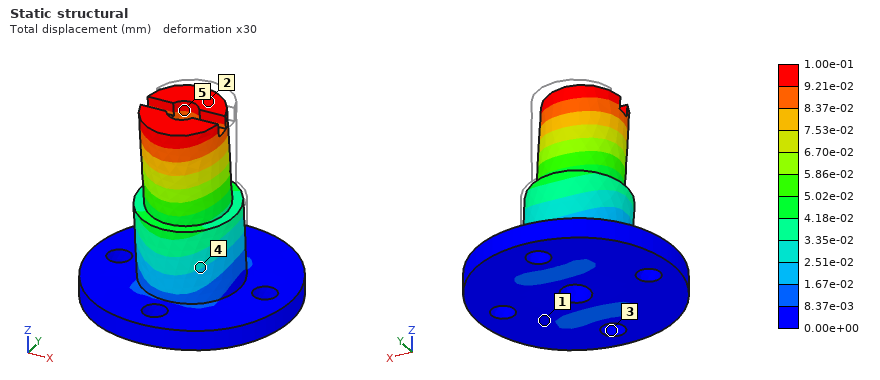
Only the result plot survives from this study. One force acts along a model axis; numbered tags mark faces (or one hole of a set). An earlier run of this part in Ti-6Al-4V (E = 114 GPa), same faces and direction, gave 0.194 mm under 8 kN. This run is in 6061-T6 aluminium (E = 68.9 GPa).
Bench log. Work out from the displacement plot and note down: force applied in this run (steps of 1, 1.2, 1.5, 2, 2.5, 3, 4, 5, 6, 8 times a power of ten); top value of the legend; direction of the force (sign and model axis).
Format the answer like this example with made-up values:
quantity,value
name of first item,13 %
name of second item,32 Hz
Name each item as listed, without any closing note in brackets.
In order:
quantity,value
force applied in this run,2.5 kN
top value of the legend,1.00e-01 mm
direction of the force,-Y
